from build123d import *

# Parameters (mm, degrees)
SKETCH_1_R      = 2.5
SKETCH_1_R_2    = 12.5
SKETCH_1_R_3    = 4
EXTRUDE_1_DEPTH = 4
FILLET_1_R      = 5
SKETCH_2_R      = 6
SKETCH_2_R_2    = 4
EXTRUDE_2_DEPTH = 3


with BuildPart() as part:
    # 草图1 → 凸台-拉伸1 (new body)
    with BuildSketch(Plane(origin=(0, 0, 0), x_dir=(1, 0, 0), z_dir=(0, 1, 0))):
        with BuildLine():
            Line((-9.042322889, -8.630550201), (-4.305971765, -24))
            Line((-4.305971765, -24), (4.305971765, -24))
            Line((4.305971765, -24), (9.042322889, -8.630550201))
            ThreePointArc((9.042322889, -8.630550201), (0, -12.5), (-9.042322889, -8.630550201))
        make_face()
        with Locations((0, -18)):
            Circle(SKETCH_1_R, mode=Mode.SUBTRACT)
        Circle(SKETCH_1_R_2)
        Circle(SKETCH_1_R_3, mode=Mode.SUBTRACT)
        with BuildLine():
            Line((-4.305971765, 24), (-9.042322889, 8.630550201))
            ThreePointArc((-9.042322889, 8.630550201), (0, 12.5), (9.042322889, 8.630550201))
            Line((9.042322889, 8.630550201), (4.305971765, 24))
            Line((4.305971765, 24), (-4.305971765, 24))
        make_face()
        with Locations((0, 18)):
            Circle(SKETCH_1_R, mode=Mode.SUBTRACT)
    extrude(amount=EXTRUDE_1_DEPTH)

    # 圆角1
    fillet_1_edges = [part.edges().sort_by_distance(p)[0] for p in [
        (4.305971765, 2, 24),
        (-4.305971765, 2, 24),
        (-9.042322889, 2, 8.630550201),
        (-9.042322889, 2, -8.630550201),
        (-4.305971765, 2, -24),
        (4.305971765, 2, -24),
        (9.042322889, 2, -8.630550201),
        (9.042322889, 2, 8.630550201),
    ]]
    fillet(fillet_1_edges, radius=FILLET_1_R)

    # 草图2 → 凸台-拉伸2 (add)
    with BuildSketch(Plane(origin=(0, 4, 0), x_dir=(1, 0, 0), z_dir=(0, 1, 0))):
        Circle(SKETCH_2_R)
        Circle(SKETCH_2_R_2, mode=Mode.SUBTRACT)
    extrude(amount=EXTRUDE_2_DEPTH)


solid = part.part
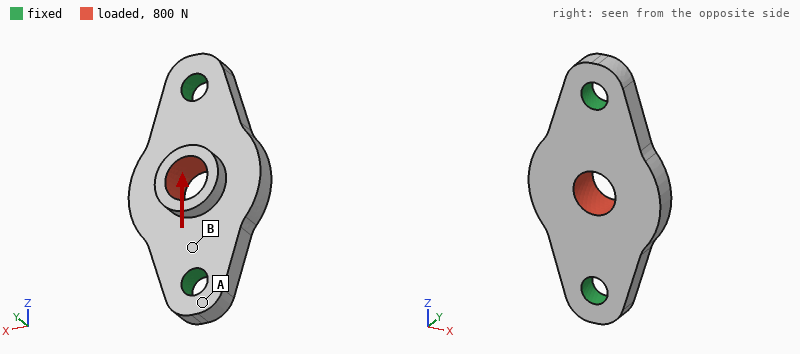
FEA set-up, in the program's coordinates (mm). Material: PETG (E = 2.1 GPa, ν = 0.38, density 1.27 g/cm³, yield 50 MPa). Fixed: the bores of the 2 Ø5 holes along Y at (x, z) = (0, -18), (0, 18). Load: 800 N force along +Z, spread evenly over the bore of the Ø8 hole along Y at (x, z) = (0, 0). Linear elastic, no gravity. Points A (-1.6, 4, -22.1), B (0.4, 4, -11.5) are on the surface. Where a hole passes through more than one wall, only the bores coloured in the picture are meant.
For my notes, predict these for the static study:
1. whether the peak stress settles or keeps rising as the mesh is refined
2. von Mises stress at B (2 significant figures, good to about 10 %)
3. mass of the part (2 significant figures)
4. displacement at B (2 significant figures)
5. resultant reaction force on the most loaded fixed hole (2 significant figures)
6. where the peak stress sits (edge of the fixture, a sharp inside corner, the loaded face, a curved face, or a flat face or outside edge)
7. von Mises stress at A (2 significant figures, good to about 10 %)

keeps rising
11 MPa
3.8 g
0.020 mm
400 N
edge of the fixture
2.2 MPa
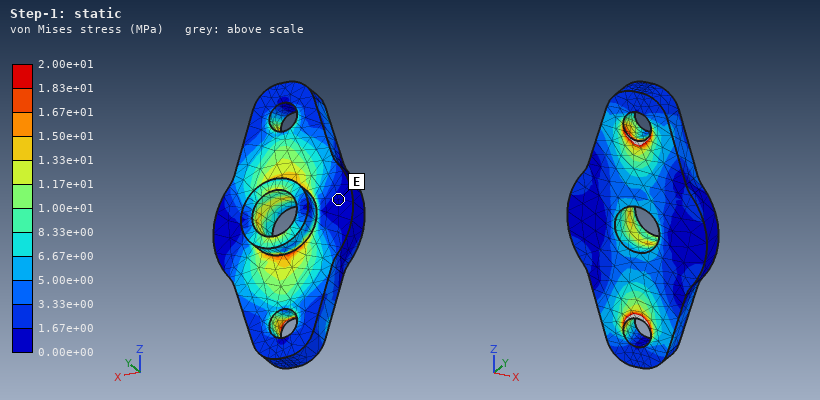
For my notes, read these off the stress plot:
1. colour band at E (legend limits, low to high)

0.00e+00 to 1.67e+00 MPa
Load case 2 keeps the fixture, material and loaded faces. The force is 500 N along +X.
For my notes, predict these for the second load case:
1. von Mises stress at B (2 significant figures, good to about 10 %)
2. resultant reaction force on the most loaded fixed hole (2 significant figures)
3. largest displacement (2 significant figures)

14 MPa
250 N
0.24 mm
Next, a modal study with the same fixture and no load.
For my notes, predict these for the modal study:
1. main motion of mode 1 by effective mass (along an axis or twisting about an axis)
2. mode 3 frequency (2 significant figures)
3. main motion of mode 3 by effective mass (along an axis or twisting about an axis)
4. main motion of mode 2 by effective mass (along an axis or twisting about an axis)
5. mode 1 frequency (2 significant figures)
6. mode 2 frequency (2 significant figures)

twisting about Z
7900 Hz
along X
along Y
3400 Hz
3600 Hz
